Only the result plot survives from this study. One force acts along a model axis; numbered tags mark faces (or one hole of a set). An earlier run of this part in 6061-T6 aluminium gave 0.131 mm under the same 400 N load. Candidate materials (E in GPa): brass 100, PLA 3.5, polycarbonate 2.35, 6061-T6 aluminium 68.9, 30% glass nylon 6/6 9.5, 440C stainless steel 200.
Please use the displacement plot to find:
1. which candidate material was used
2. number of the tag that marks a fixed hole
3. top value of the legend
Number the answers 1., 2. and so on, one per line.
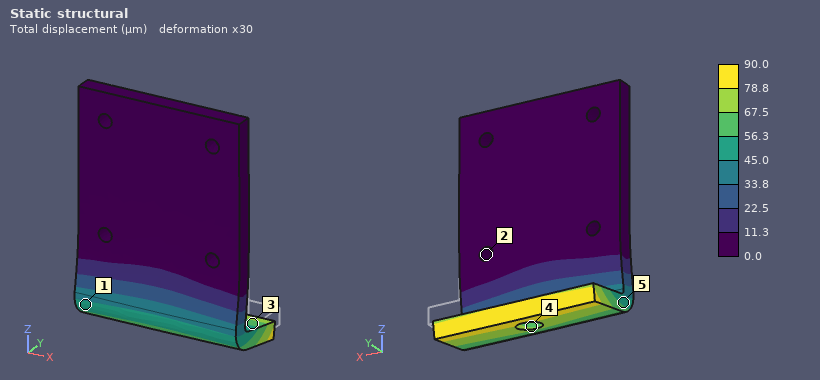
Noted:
1. brass
2. 2
3. 90.0 µm
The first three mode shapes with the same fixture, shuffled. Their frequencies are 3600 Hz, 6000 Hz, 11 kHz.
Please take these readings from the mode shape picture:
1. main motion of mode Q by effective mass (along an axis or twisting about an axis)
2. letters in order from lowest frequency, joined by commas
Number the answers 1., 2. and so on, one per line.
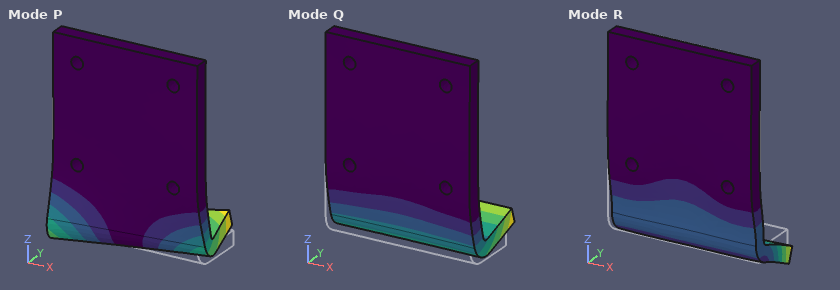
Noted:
1. along Y
2. Q, P, R
